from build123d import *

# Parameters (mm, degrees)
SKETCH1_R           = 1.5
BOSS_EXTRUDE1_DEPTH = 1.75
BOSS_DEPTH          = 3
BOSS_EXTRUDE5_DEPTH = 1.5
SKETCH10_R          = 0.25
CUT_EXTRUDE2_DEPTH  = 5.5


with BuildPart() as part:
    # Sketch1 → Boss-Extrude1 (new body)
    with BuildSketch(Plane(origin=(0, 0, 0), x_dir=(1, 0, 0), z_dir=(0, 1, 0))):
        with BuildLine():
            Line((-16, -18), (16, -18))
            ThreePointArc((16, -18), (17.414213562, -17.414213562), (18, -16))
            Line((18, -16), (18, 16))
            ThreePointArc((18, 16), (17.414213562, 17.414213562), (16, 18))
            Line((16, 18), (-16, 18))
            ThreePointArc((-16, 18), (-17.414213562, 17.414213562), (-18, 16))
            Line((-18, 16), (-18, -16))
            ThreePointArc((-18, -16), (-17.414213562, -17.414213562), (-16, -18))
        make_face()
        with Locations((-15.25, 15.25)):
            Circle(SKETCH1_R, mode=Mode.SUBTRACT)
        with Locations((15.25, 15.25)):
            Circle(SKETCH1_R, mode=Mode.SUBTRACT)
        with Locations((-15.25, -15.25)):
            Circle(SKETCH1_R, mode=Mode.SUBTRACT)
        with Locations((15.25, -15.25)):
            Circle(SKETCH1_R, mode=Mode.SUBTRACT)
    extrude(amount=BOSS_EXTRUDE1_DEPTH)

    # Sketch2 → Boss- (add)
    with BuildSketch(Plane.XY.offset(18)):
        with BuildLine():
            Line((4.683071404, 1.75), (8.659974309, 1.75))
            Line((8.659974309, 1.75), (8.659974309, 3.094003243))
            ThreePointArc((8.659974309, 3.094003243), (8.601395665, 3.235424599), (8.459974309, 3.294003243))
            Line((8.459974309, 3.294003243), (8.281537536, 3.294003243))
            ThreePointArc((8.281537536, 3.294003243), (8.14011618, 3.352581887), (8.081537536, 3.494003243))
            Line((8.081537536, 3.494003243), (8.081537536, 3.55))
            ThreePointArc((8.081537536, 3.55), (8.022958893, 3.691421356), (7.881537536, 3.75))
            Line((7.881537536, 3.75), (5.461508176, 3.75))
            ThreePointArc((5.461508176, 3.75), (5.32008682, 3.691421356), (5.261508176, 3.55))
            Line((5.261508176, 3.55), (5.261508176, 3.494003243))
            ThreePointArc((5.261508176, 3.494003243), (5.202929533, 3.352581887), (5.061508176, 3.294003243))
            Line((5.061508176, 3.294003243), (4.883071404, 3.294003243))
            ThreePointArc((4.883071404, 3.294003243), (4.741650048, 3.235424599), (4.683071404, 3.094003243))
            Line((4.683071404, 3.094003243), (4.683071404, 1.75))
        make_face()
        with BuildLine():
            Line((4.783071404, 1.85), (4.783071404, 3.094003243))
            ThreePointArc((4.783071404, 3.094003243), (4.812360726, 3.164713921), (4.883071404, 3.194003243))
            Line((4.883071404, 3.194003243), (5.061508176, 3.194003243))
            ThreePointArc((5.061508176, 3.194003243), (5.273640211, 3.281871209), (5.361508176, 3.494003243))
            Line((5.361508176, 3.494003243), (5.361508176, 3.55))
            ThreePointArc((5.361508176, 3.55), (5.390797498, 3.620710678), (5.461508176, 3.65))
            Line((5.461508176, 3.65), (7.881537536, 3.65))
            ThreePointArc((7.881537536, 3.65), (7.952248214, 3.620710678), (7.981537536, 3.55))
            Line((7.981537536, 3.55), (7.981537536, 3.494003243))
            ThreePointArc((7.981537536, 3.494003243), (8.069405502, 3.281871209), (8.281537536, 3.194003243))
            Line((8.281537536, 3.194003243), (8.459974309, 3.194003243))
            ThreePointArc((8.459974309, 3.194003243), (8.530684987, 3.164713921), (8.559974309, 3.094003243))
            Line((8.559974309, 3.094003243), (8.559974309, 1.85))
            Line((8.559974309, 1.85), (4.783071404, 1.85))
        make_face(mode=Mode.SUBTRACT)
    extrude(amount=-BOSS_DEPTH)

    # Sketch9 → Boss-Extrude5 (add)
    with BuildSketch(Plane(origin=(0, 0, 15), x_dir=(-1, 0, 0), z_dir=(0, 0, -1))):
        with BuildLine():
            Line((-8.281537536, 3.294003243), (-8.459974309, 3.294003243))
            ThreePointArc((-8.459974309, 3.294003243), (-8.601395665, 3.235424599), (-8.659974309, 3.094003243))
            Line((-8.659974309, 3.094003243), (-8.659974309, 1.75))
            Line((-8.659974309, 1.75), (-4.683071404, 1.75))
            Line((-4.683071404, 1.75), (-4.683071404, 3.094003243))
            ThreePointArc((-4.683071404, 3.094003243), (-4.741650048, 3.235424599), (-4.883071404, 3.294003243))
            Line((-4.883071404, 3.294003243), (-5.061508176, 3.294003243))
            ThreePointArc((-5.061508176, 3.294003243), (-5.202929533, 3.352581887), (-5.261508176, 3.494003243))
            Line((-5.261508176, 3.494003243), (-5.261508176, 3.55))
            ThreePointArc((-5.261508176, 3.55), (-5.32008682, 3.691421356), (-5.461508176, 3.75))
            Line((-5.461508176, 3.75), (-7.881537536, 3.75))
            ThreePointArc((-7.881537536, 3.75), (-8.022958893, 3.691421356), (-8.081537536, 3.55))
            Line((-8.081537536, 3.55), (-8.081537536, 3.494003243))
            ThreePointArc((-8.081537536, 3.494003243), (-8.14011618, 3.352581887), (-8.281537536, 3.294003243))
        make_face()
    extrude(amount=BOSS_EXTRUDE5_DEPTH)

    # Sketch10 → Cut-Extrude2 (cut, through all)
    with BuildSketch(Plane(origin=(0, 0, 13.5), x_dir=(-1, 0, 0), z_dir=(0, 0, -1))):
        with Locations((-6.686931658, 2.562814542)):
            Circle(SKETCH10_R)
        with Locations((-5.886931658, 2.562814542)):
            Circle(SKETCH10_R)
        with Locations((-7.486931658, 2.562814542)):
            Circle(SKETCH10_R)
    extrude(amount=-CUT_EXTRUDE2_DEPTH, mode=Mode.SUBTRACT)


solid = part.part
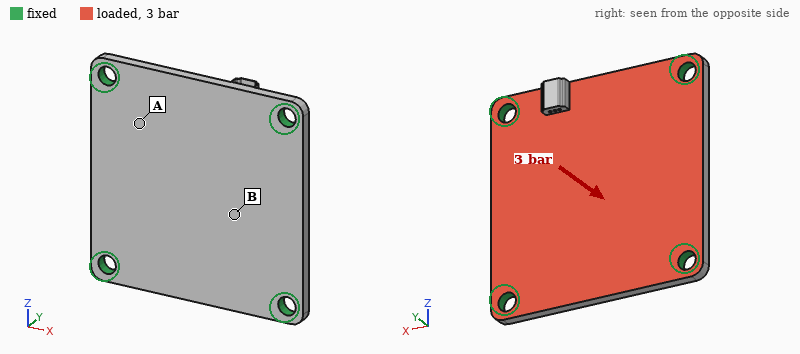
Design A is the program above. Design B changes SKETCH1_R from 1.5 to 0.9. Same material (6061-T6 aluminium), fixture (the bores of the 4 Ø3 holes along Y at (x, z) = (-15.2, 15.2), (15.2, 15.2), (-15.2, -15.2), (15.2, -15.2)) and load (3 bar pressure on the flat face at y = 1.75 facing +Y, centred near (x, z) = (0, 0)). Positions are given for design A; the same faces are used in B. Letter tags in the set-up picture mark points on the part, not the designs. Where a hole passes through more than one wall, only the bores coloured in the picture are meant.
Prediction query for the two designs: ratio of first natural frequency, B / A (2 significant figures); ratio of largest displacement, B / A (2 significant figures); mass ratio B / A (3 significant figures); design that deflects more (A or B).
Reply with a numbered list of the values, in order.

1. 0.90
2. 1.2
3. 1.01
4. B
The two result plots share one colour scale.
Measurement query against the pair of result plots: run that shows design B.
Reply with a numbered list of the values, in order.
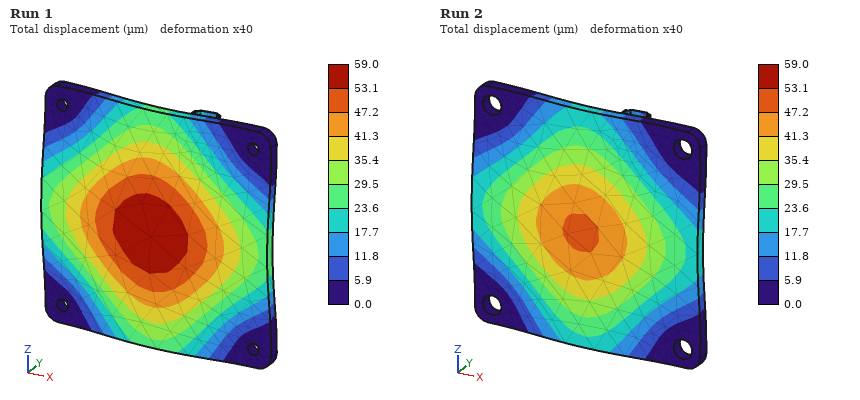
1. Run 1
